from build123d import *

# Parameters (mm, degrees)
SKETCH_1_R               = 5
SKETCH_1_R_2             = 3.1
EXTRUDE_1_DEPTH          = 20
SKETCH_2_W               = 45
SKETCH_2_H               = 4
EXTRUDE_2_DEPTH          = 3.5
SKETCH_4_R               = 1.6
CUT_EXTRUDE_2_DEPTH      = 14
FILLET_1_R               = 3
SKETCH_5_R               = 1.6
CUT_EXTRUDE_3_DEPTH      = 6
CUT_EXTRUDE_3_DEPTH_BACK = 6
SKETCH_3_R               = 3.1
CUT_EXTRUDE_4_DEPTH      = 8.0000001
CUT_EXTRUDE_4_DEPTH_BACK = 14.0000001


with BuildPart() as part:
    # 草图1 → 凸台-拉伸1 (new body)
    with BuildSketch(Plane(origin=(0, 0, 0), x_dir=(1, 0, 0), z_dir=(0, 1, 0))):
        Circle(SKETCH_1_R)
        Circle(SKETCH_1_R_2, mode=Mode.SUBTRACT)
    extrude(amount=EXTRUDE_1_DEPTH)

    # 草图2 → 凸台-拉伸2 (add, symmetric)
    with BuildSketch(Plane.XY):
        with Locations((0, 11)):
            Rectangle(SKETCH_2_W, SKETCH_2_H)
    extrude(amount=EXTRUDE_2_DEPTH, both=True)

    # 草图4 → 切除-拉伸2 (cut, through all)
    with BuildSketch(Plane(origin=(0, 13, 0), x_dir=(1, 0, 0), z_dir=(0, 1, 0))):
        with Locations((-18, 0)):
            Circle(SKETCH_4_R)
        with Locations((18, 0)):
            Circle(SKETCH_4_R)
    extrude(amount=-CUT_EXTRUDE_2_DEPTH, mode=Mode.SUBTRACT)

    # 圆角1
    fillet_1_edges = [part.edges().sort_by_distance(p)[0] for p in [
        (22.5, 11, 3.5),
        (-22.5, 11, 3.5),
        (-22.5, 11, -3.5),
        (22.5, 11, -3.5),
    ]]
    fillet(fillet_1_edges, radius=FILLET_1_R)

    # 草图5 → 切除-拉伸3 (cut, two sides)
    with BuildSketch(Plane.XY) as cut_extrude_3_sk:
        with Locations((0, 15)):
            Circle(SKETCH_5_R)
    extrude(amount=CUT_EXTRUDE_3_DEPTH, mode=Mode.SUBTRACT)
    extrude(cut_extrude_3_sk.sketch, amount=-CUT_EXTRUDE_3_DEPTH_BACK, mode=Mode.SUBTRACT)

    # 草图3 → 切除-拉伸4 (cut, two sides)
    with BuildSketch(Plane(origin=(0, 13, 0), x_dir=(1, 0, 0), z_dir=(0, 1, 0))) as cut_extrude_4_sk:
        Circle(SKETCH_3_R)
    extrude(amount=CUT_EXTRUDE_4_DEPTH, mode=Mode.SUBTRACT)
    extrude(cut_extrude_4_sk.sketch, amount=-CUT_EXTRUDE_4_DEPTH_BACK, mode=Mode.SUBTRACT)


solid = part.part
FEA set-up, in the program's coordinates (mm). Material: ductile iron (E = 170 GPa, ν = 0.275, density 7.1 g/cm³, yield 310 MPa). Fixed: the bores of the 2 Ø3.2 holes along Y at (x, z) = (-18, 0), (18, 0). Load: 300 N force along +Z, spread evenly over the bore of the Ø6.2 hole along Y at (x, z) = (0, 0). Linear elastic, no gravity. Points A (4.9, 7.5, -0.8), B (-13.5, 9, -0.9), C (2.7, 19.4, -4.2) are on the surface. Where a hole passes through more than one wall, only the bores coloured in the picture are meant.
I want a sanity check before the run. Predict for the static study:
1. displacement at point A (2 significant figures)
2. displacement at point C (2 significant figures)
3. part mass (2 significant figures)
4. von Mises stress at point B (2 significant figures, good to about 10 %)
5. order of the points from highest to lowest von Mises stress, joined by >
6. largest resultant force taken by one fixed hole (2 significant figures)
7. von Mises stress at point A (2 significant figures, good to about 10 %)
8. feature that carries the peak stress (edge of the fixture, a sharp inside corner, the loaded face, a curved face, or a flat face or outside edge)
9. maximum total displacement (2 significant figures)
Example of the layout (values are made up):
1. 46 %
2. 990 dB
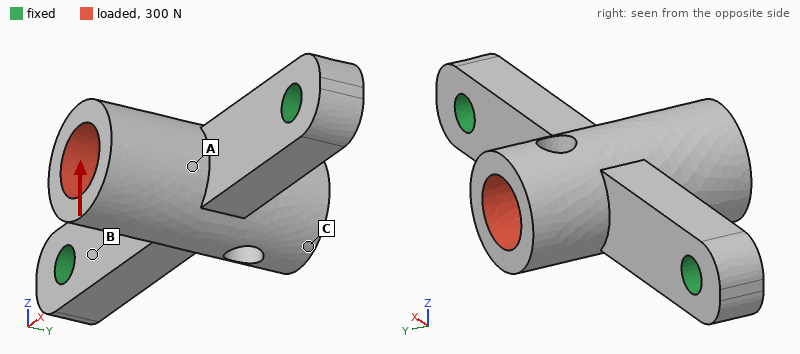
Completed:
1. 5.7 µm
2. 2.2 µm
3. 13 g
4. 24 MPa
5. B > A > C
6. 150 N
7. 14 MPa
8. edge of the fixture
9. 9.6 µm
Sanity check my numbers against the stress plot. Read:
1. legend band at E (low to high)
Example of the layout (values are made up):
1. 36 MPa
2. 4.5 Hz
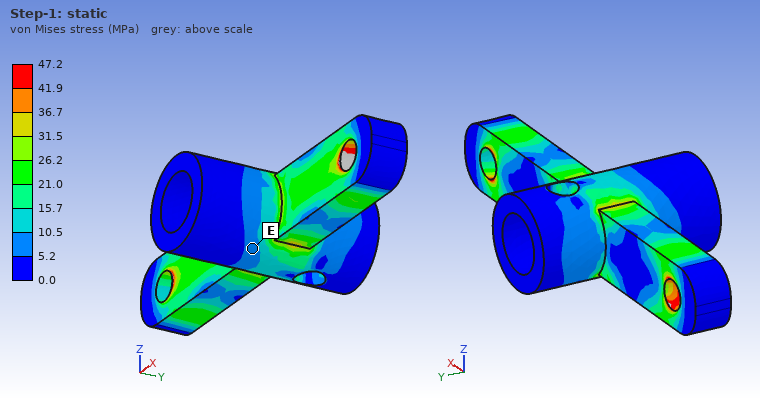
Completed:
1. 5.2 to 10.5 MPa
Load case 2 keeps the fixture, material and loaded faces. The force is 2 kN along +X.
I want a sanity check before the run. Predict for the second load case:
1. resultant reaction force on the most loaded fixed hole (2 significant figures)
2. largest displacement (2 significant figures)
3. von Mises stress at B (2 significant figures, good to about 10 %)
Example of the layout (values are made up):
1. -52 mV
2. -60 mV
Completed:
1. 1.0 kN
2. 13 µm
3. 31 MPa
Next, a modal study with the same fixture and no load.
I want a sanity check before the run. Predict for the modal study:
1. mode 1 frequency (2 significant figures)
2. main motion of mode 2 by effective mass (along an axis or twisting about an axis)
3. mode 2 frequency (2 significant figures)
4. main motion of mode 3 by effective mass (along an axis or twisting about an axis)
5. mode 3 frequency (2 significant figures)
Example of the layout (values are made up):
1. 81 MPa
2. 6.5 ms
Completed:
1. 9100 Hz
2. along Y
3. 11 kHz
4. along Z
5. 15 kHz
